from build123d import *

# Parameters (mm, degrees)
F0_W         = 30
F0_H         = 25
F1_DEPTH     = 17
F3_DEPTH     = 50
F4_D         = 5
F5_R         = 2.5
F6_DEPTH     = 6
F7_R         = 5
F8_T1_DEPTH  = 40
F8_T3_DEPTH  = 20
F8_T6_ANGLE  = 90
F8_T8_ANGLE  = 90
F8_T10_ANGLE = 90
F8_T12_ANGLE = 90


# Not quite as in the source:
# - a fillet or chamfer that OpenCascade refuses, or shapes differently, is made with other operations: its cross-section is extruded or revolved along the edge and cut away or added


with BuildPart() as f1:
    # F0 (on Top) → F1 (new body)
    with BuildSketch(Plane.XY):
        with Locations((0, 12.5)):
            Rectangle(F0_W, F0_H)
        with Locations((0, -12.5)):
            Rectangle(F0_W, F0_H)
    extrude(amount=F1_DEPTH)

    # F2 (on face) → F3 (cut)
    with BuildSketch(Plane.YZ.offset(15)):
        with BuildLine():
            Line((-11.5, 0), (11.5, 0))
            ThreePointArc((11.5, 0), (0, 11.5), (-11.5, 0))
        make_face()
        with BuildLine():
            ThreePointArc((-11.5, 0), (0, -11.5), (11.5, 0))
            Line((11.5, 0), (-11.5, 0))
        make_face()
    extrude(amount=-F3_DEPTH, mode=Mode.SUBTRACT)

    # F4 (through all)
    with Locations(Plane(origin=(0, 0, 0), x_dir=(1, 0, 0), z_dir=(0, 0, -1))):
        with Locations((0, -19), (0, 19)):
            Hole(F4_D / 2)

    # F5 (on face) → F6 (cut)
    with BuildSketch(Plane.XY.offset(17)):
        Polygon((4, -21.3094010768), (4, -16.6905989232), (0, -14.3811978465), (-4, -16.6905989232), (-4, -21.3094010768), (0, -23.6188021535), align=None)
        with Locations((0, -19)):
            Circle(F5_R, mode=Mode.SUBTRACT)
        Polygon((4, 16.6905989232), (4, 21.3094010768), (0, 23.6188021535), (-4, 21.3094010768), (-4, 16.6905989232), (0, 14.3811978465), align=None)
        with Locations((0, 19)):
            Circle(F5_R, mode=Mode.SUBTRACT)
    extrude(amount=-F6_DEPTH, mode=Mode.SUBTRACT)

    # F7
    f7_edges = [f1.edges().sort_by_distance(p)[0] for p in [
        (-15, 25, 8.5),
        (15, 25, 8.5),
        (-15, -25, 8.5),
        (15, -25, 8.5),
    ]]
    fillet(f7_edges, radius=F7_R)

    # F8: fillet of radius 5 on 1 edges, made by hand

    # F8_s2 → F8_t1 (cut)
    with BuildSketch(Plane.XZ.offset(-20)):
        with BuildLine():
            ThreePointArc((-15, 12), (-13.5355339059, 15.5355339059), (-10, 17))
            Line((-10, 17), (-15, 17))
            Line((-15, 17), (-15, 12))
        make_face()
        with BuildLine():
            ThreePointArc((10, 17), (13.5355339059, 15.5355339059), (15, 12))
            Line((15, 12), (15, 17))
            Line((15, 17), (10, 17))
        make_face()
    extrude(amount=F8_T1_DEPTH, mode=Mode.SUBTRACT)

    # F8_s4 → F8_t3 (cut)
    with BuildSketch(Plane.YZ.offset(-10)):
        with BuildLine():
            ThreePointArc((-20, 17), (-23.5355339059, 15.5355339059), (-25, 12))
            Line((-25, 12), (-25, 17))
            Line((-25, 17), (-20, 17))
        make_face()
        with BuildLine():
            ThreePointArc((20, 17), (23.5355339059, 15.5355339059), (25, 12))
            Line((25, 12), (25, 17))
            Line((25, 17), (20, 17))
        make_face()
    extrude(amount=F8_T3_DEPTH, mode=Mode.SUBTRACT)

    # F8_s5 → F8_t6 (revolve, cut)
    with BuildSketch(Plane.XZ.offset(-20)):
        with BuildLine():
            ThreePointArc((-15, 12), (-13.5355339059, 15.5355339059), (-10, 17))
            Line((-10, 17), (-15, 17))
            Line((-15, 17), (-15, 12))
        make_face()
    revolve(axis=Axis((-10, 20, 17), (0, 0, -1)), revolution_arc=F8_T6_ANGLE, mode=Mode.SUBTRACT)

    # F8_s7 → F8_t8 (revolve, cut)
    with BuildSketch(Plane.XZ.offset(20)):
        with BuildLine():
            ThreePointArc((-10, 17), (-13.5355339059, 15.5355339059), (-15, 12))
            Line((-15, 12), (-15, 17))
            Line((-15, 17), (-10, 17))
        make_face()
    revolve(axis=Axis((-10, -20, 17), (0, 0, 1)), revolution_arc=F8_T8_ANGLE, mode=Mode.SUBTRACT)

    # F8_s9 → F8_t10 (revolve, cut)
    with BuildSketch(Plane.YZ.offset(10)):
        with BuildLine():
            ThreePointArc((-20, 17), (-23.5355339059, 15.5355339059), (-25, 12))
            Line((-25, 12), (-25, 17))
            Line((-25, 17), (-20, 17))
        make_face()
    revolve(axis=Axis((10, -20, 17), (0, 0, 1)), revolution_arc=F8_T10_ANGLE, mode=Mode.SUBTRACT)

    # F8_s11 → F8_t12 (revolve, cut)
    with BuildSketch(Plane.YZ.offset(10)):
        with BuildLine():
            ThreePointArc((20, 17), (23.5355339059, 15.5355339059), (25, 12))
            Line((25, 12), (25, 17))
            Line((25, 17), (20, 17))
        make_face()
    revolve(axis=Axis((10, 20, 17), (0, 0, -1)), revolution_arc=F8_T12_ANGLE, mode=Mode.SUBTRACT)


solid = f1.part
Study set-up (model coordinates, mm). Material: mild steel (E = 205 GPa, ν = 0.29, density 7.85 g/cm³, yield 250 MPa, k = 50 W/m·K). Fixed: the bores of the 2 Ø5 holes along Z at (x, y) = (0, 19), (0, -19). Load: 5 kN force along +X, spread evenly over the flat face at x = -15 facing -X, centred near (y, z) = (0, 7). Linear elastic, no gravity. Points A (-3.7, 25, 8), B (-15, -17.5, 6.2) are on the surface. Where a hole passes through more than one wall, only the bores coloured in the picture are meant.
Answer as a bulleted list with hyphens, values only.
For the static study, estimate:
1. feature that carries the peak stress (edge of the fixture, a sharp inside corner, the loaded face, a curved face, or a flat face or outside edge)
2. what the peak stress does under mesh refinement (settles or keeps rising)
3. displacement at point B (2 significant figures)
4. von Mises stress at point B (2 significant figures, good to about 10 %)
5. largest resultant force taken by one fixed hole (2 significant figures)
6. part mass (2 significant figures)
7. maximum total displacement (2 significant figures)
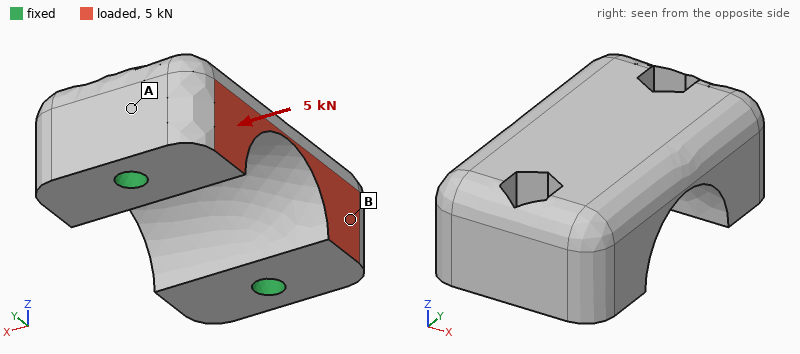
- edge of the fixture
- keeps rising
- 1.7 µm
- 14 MPa
- 2.5 kN
- 130 g
- 2.4 µm
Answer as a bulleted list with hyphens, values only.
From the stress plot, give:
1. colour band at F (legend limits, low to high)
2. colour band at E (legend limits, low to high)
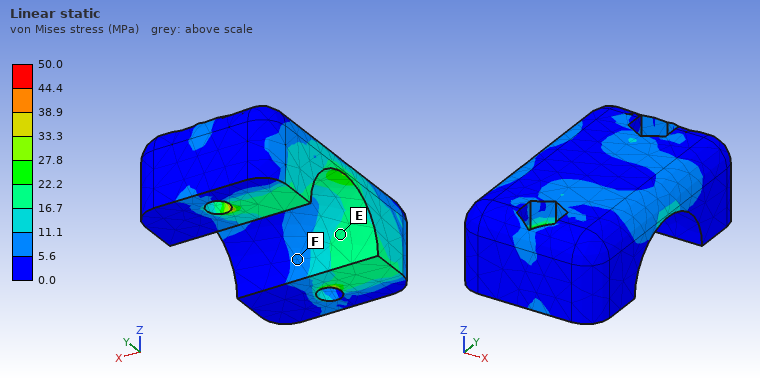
- 5.6 to 11.1 MPa
- 16.7 to 22.2 MPa
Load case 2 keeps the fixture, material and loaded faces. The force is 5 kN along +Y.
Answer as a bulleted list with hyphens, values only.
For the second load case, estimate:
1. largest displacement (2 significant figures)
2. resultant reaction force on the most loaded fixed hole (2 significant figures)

- 6.9 µm
- 2.9 kN
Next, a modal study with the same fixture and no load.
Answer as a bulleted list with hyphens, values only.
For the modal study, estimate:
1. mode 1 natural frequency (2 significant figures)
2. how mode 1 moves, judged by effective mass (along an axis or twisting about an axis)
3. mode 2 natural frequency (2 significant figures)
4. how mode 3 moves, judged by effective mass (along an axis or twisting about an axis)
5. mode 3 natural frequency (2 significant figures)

- 18 kHz
- along X
- 25 kHz
- along Z
- 27 kHz
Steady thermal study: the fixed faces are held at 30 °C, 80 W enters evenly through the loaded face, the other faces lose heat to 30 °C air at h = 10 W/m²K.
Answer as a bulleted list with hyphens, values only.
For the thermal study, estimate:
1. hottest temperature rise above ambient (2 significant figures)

- 64 K
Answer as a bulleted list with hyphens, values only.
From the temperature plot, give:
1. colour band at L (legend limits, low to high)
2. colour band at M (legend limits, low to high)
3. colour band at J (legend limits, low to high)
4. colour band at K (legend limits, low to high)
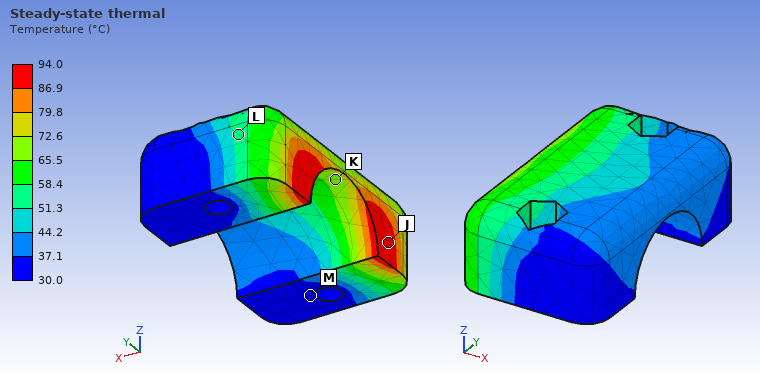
- 51.3 to 58.4 °C
- 30.0 to 37.1 °C
- 86.9 to 94.0 °C
- 65.5 to 72.6 °C
